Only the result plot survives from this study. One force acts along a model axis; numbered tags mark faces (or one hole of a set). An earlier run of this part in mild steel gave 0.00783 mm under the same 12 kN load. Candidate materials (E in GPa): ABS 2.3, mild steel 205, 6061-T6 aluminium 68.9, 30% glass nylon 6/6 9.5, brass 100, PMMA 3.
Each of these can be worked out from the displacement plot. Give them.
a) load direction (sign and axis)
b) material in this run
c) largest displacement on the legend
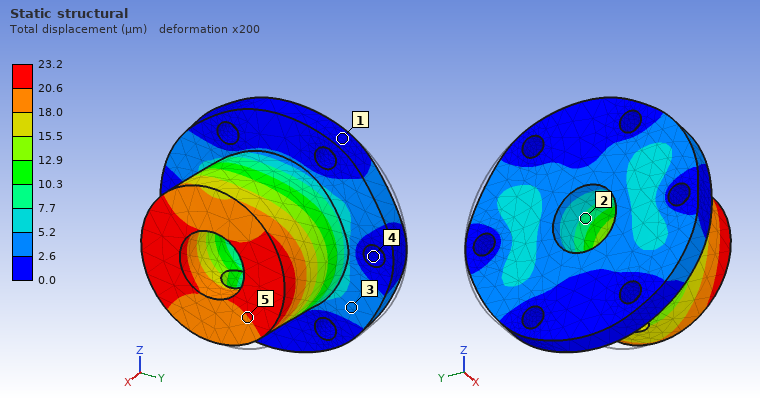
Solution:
-Y
6061-T6 aluminium
23.2 µm
